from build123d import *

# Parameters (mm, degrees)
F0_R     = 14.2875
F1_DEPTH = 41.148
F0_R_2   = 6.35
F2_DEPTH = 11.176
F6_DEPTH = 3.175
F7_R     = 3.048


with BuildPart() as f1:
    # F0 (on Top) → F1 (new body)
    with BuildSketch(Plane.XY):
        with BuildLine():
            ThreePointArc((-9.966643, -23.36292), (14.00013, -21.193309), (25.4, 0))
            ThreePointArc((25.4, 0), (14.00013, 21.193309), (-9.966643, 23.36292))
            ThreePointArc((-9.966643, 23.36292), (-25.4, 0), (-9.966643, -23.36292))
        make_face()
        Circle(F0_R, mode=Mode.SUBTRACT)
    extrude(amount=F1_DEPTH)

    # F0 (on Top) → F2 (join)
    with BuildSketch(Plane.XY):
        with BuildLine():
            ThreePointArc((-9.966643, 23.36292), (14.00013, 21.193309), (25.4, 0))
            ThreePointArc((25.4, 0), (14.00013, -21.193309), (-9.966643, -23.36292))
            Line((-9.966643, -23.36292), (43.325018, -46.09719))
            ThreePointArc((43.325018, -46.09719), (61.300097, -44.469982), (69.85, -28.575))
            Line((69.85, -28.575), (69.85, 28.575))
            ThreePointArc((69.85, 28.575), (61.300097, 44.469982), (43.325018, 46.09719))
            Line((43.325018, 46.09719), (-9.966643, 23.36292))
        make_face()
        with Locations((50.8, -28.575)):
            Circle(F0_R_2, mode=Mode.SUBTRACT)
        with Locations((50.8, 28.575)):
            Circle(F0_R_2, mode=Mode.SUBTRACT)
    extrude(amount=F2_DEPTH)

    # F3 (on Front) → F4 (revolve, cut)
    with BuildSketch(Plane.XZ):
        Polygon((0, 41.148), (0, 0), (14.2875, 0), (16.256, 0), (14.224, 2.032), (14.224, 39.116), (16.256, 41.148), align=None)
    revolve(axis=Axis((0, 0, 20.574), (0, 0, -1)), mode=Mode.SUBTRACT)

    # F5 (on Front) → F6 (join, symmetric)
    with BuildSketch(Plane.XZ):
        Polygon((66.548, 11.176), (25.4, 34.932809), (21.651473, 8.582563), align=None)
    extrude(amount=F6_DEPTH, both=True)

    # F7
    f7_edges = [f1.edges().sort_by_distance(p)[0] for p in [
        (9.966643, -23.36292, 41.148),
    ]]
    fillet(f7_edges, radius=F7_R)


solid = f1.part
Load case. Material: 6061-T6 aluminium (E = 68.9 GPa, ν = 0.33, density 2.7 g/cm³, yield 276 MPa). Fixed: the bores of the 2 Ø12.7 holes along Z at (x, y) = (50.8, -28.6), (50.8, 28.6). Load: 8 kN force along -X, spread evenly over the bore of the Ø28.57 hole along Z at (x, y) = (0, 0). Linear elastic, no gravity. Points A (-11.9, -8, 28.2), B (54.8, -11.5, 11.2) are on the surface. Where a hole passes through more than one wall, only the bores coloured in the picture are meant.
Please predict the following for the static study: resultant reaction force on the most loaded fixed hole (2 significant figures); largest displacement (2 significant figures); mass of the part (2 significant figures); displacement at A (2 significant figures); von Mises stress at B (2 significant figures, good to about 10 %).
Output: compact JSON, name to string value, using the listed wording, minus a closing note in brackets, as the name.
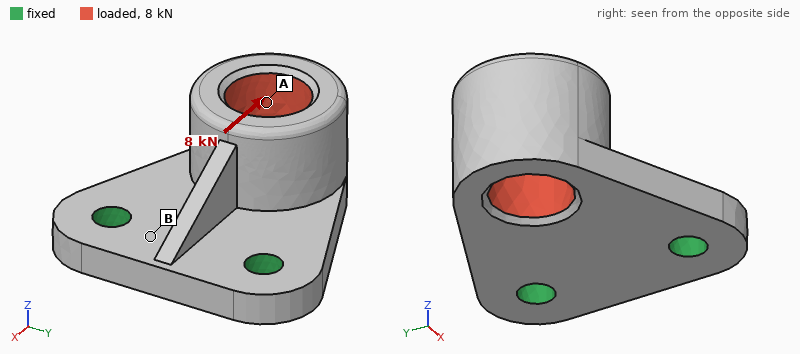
{"resultant reaction force on the most loaded fixed hole": "4.1 kN", "largest displacement": "0.24 mm", "mass of the part": "290 g", "displacement at A": "0.18 mm", "von Mises stress at B": "28 MPa"}
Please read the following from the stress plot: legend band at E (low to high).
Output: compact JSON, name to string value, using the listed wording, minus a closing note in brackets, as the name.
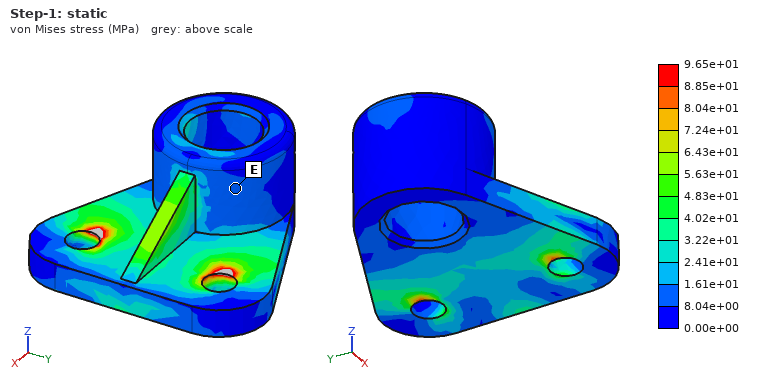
{"legend band at E": "8.04e+00 to 1.61e+01 MPa"}
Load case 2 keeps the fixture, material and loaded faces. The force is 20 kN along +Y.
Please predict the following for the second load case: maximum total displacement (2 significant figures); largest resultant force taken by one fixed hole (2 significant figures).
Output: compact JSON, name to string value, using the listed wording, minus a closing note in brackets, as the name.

{"maximum total displacement": "0.25 mm", "largest resultant force taken by one fixed hole": "19 kN"}
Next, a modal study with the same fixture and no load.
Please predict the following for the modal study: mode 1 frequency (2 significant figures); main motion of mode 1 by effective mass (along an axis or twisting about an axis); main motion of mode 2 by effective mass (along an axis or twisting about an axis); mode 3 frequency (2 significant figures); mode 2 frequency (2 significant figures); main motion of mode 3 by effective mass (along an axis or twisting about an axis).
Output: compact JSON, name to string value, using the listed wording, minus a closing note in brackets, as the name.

{"mode 1 frequency": "1700 Hz", "main motion of mode 1 by effective mass": "along Z", "main motion of mode 2 by effective mass": "along Y", "mode 3 frequency": "6900 Hz", "mode 2 frequency": "3900 Hz", "main motion of mode 3 by effective mass": "along Y"}
